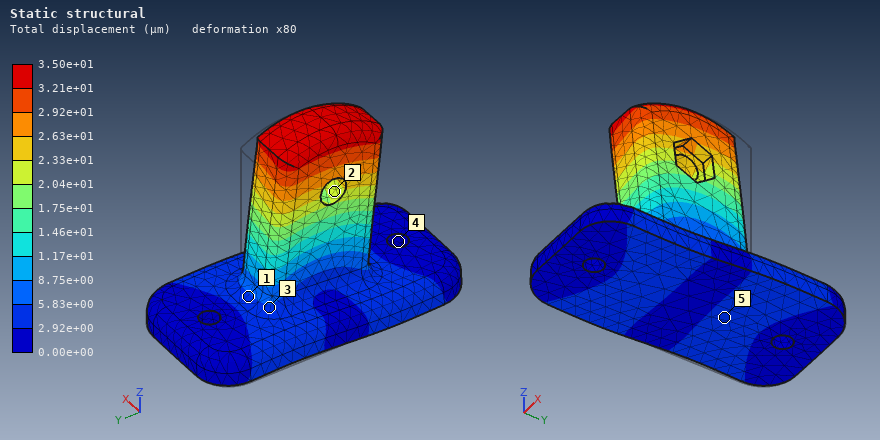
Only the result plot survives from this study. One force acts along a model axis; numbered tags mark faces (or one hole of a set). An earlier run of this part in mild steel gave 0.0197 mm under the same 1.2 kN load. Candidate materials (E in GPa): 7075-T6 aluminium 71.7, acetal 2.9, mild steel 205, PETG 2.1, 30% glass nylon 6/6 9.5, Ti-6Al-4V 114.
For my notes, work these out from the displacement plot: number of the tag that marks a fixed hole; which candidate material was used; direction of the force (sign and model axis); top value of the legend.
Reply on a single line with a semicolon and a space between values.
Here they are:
4; Ti-6Al-4V; -Y; 3.50e+01 µm
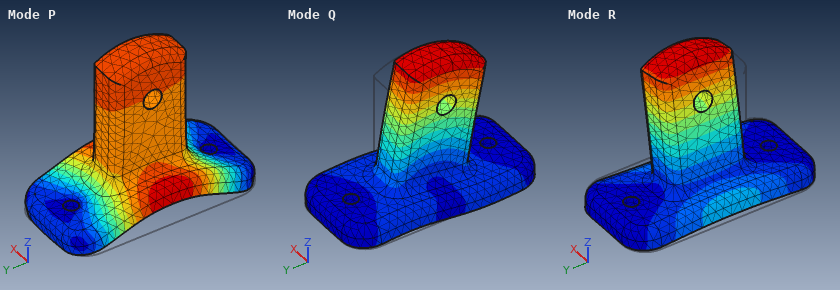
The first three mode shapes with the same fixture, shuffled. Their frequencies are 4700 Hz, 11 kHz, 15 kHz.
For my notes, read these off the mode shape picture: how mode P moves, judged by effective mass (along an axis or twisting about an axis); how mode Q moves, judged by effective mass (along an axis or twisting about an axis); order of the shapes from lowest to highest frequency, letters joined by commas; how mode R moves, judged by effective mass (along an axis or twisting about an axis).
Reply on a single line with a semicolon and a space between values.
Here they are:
along Z; along Y; R, Q, P; along X
